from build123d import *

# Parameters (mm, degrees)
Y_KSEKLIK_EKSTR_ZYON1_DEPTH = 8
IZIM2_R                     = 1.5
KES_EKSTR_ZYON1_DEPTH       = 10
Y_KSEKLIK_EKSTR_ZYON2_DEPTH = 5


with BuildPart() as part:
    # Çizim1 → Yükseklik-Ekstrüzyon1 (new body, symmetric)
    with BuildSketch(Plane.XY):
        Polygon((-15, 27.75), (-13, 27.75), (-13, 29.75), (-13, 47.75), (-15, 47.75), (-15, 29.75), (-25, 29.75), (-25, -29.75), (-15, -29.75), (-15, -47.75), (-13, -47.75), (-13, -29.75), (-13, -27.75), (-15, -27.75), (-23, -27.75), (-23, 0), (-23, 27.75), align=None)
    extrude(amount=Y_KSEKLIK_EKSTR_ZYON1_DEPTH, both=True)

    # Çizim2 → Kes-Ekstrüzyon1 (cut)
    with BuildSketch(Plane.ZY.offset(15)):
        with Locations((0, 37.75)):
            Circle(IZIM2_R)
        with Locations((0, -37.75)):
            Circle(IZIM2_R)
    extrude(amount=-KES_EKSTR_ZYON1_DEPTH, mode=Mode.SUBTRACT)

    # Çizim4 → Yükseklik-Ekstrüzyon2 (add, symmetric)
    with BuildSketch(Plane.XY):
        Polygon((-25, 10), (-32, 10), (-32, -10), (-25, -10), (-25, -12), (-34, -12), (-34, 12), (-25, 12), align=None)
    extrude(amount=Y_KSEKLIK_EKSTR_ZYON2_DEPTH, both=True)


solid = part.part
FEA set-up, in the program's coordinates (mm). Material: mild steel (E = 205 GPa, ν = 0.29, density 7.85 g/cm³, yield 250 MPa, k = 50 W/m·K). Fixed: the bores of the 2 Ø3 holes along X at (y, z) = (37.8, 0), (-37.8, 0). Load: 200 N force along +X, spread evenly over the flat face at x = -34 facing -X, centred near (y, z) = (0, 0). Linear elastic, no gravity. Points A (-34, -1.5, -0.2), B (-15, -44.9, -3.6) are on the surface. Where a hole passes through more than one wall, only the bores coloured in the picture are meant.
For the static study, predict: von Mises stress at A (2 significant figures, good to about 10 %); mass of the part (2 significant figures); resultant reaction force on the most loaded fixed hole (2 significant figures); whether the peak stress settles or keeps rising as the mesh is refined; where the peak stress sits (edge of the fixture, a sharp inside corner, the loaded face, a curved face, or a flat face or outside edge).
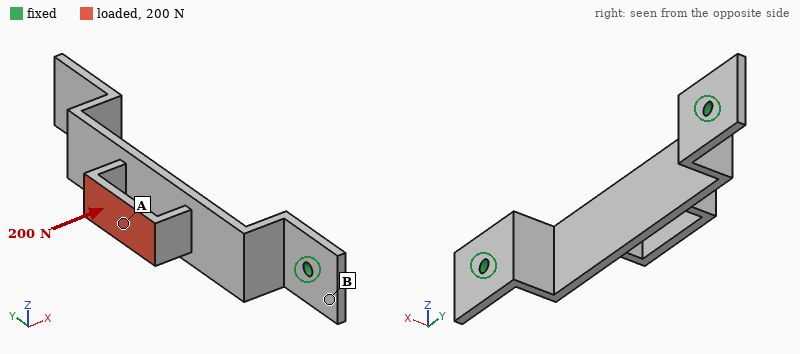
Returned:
25 MPa
35 g
170 N
keeps rising
edge of the fixture
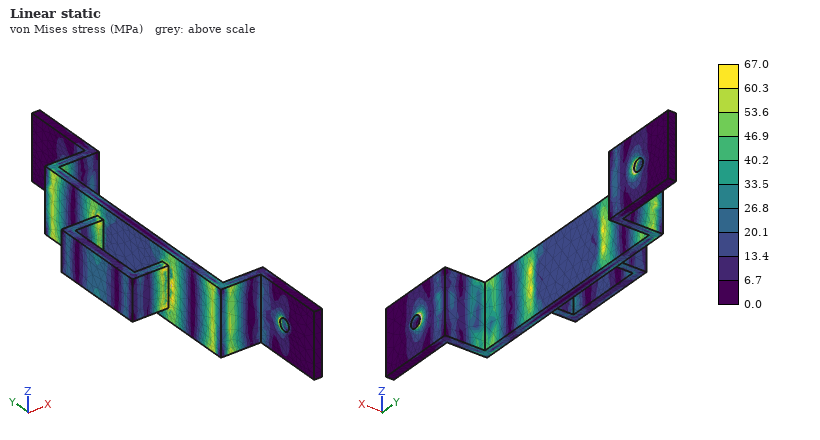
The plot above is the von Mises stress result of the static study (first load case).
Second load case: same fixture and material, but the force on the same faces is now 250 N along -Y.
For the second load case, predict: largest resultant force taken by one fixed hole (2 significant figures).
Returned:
140 N
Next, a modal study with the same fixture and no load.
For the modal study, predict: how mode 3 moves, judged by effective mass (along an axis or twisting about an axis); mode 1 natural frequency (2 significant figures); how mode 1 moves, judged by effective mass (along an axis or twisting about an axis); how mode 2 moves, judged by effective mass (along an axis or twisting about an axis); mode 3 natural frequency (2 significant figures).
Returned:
along Y
2200 Hz
along Z
along X
3000 Hz
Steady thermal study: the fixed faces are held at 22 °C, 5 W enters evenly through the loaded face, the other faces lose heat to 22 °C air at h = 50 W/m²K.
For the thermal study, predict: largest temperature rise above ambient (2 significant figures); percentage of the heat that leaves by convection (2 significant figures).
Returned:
49 K
69 %
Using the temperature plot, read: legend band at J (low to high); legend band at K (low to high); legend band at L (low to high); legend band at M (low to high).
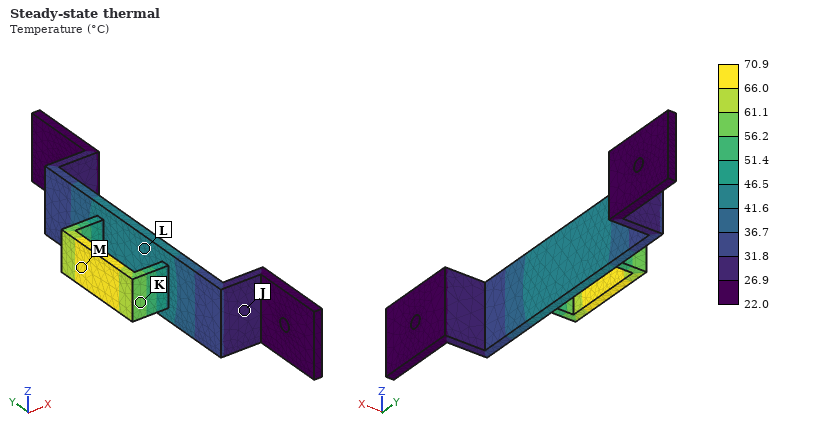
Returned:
26.9 to 31.8 °C
56.2 to 61.1 °C
41.6 to 46.5 °C
66.0 to 70.9 °C
